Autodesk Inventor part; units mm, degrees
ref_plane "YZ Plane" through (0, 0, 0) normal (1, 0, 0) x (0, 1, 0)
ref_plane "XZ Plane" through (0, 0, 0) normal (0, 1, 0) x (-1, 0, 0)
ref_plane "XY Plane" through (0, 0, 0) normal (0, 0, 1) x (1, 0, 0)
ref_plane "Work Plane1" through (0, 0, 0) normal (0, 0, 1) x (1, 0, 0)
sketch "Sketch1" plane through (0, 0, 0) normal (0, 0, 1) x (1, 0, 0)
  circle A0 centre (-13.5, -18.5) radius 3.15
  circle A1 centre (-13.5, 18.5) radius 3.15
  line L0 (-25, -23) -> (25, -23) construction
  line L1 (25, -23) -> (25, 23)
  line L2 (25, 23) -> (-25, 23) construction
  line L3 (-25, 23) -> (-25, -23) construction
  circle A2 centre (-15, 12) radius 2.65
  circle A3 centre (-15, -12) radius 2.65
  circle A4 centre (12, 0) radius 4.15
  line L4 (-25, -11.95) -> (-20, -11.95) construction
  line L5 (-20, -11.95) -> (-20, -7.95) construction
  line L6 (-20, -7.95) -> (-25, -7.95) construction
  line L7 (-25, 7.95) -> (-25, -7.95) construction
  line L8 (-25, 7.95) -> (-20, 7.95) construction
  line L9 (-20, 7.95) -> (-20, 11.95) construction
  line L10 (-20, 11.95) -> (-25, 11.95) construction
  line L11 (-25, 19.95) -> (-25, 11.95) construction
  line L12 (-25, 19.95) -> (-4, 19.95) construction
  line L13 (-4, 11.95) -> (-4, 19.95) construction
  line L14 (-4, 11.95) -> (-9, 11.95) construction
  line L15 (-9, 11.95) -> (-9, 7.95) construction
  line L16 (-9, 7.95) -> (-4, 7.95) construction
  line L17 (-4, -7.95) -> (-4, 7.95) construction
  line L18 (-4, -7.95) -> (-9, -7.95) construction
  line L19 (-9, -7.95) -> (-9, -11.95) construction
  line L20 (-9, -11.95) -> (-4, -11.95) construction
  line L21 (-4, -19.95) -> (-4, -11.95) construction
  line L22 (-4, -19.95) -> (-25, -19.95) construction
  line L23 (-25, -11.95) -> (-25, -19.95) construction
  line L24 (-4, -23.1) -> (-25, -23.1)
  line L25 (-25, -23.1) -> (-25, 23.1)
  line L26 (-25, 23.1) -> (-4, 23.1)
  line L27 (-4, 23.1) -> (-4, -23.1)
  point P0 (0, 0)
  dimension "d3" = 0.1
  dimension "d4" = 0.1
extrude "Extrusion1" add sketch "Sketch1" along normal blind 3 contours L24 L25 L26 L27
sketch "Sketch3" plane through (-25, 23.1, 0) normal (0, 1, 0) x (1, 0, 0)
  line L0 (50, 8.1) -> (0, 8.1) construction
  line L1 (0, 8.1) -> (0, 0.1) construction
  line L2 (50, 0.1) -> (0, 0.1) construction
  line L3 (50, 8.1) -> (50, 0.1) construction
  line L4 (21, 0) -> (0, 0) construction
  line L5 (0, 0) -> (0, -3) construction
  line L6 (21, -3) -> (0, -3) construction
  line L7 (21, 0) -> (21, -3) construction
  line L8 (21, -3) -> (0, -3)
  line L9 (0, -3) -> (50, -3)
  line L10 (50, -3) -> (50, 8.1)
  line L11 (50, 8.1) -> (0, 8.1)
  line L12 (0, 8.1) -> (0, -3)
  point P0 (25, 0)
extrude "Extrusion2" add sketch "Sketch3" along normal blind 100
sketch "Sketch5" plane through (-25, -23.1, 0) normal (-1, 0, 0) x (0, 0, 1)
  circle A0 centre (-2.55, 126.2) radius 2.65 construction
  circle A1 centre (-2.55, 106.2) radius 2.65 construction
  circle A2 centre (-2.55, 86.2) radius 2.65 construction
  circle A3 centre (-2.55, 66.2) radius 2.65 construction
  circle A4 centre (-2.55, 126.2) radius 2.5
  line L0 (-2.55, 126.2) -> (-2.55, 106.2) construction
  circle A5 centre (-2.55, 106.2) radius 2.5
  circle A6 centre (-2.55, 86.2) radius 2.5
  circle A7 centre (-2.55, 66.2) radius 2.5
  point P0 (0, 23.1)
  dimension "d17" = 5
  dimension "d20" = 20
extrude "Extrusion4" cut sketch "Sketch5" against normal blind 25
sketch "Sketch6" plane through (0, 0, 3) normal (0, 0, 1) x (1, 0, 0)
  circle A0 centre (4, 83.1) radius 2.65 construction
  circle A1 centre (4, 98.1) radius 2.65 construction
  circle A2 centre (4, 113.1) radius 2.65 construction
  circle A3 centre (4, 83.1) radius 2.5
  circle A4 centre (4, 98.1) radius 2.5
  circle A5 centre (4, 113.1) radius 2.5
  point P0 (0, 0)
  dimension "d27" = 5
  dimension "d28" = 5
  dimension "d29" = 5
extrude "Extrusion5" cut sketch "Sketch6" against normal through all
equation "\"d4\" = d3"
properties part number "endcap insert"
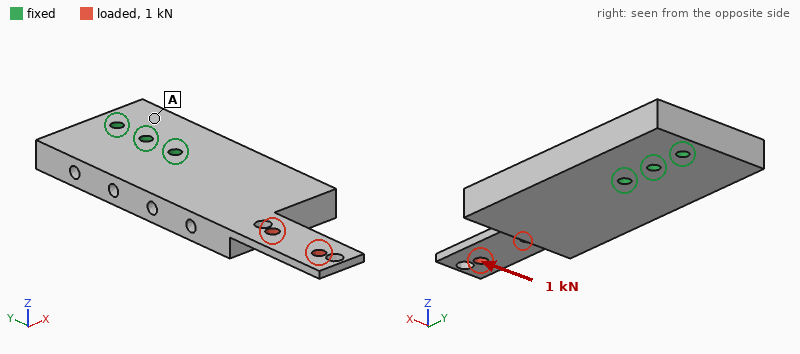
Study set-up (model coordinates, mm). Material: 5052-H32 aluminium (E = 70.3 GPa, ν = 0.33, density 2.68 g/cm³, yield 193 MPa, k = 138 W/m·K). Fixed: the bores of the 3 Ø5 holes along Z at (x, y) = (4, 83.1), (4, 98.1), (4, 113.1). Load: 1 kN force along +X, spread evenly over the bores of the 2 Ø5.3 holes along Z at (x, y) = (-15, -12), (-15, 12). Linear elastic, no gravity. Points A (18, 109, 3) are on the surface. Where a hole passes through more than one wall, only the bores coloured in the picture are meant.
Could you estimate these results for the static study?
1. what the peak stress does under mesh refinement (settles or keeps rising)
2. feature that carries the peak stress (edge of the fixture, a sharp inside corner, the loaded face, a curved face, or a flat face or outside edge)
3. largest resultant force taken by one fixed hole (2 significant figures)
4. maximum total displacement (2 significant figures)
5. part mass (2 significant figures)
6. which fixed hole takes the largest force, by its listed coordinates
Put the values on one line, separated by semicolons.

keeps rising; a sharp inside corner; 3.5 kN; 0.25 mm; 150 g; (4, 83.1)
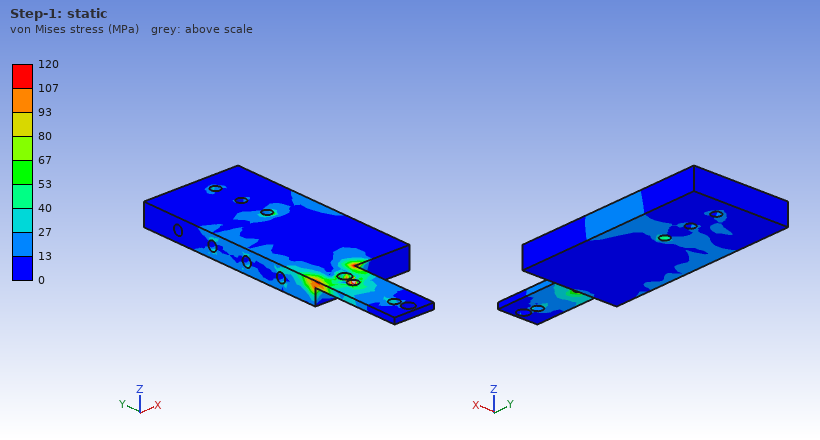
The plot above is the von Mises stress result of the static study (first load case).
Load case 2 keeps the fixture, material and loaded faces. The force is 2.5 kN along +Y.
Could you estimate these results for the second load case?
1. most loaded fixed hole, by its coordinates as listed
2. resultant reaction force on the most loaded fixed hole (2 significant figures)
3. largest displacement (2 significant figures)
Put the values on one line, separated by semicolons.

(4, 83.1); 2.2 kN; 0.19 mm
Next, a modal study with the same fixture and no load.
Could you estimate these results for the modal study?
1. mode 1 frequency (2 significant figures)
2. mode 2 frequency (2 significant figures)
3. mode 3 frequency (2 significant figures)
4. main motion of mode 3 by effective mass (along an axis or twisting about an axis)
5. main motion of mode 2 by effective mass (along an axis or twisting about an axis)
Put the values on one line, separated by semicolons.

970 Hz; 2200 Hz; 3800 Hz; along X; along Z
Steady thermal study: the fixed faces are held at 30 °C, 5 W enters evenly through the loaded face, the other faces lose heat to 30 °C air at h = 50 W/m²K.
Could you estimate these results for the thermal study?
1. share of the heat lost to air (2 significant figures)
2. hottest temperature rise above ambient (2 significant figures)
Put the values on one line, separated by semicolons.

42 %; 17 K
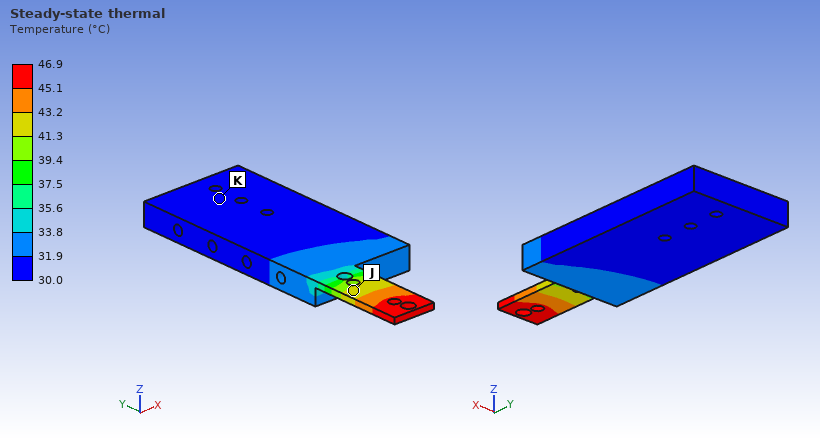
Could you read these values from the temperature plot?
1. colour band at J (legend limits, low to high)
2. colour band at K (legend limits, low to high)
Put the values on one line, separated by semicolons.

41.3 to 43.2 °C; 30.0 to 31.9 °C
